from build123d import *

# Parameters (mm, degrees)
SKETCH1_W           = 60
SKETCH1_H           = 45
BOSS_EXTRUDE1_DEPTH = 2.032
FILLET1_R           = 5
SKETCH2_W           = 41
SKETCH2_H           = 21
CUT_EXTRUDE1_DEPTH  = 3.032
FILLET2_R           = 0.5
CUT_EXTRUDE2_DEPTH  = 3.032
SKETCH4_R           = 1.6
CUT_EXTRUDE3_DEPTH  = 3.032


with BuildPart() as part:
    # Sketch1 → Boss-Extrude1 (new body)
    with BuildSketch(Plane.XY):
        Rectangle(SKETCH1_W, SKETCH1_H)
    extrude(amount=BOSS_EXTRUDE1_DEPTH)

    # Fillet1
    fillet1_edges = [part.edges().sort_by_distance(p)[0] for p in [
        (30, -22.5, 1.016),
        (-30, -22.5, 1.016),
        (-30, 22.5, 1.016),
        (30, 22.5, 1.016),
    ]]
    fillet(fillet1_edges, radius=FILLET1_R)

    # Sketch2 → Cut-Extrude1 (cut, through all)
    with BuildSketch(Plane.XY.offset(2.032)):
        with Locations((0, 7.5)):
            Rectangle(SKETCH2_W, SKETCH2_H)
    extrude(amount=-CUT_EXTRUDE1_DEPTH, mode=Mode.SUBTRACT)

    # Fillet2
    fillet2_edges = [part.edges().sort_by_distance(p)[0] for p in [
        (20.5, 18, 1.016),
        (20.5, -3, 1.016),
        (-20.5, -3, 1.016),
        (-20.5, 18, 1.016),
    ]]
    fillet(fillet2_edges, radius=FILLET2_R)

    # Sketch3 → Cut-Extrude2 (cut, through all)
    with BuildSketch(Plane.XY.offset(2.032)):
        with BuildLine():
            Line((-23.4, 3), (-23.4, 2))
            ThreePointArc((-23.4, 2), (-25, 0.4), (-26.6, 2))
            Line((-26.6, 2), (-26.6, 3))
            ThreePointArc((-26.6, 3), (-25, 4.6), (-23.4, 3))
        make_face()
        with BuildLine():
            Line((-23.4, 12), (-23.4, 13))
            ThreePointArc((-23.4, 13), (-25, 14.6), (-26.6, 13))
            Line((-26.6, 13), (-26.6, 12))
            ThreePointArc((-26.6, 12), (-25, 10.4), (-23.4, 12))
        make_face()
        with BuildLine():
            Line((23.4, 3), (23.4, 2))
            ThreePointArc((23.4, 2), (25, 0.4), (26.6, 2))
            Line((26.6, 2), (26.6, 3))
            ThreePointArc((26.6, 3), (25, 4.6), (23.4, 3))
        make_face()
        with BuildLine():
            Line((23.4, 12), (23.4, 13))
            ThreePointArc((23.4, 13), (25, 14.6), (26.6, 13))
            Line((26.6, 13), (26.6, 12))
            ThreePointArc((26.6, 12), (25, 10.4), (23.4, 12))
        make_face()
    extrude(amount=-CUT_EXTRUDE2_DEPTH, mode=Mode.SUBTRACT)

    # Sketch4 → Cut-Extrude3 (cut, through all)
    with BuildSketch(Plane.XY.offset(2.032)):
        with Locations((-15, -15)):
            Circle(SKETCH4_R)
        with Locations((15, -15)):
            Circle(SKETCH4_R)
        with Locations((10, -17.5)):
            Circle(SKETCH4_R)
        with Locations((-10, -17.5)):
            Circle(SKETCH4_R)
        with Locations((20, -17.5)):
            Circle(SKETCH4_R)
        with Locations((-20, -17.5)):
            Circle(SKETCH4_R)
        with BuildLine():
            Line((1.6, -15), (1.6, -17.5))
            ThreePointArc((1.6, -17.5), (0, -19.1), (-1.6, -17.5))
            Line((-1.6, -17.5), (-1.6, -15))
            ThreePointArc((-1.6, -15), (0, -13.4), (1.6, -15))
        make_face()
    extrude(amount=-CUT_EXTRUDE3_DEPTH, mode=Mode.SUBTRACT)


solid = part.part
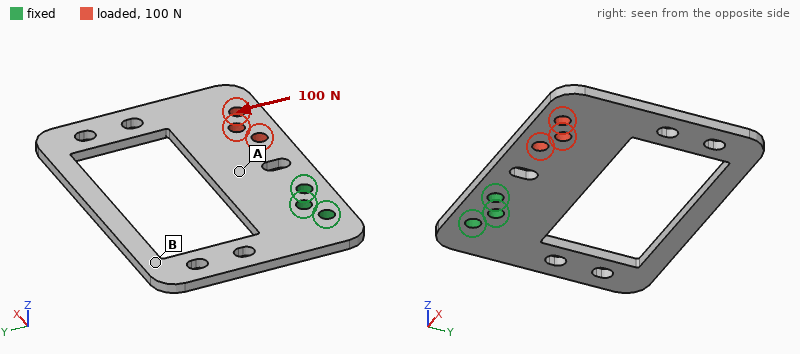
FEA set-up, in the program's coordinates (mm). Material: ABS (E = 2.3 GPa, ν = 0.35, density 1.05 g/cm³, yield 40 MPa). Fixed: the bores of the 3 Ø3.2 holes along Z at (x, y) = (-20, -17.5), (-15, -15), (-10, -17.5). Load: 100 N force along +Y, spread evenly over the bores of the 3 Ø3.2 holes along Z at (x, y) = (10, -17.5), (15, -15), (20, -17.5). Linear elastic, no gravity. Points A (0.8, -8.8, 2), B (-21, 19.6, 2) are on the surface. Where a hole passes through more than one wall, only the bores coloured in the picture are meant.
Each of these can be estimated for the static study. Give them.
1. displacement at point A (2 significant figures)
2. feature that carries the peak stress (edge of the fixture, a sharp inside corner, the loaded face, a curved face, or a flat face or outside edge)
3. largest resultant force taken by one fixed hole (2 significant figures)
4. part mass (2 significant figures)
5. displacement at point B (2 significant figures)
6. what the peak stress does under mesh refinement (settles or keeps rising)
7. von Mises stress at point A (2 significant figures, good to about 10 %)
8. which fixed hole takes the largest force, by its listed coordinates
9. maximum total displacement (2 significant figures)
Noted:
0.21 mm
edge of the fixture
260 N
3.6 g
0.41 mm
keeps rising
8.1 MPa
(-10, -17.5)
0.82 mm
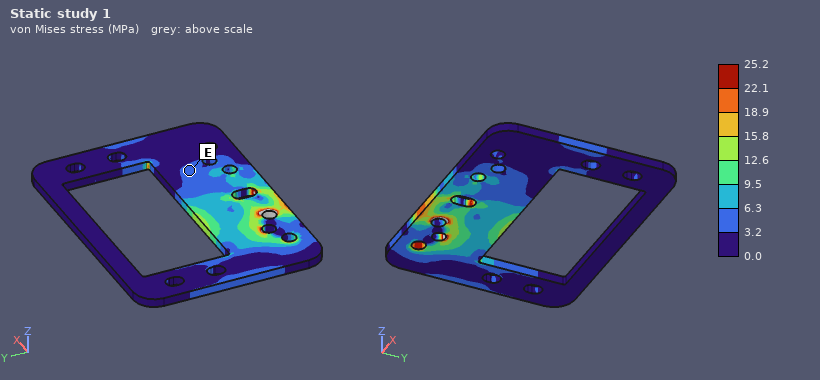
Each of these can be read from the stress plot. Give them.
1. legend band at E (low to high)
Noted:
3.2 to 6.3 MPa
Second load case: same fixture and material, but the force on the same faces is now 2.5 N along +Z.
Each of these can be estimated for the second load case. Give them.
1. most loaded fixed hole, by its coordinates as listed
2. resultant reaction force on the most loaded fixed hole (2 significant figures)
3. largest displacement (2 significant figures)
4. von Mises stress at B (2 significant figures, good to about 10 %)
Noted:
(-10, -17.5)
5.7 N
0.85 mm
0.83 MPa
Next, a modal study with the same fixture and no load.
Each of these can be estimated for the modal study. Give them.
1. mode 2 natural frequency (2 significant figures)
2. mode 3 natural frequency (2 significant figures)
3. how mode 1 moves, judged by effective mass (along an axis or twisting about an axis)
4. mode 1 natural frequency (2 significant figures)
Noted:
310 Hz
520 Hz
along Z
180 Hz
